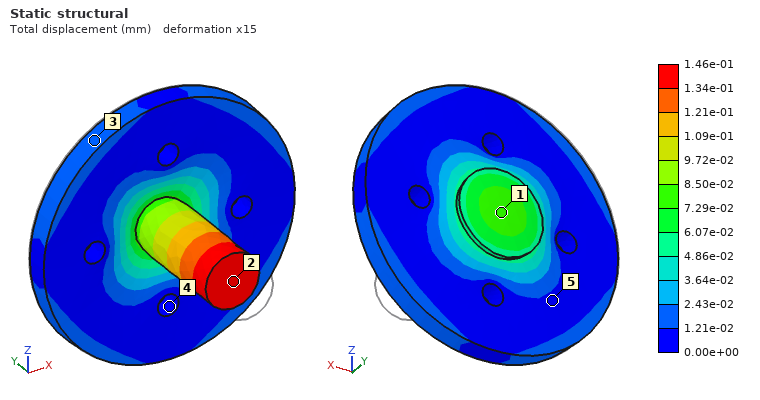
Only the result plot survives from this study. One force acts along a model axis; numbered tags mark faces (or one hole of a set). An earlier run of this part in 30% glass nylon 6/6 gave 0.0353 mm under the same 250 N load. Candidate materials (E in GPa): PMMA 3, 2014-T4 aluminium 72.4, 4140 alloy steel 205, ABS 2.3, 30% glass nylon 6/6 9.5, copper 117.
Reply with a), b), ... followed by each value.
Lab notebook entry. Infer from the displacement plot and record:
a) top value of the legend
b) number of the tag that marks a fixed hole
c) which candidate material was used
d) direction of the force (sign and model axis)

a) 1.46e-01 mm
b) 4
c) ABS
d) +Y
